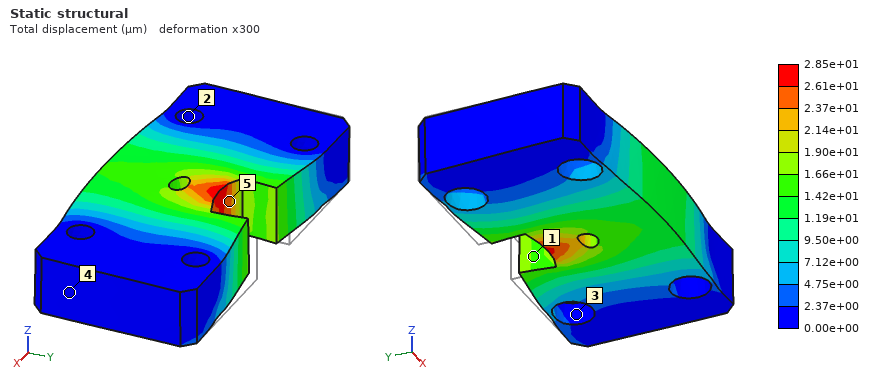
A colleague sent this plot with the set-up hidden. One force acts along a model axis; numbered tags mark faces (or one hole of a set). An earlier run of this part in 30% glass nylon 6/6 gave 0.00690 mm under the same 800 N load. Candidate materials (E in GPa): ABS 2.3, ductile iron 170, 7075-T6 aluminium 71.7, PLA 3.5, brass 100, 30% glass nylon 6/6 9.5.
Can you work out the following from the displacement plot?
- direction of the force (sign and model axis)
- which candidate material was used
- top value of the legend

-Y
ABS
2.85e+01 µm
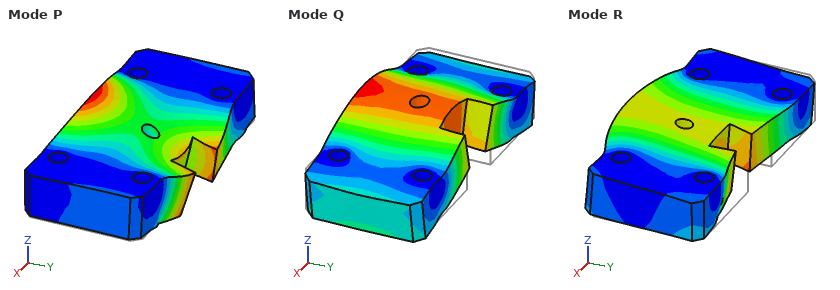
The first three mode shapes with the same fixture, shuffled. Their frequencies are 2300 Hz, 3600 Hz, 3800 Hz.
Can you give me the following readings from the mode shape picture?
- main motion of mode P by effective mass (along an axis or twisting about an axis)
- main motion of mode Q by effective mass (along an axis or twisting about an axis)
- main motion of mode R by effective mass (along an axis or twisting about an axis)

twisting about X
along Z
along Y
